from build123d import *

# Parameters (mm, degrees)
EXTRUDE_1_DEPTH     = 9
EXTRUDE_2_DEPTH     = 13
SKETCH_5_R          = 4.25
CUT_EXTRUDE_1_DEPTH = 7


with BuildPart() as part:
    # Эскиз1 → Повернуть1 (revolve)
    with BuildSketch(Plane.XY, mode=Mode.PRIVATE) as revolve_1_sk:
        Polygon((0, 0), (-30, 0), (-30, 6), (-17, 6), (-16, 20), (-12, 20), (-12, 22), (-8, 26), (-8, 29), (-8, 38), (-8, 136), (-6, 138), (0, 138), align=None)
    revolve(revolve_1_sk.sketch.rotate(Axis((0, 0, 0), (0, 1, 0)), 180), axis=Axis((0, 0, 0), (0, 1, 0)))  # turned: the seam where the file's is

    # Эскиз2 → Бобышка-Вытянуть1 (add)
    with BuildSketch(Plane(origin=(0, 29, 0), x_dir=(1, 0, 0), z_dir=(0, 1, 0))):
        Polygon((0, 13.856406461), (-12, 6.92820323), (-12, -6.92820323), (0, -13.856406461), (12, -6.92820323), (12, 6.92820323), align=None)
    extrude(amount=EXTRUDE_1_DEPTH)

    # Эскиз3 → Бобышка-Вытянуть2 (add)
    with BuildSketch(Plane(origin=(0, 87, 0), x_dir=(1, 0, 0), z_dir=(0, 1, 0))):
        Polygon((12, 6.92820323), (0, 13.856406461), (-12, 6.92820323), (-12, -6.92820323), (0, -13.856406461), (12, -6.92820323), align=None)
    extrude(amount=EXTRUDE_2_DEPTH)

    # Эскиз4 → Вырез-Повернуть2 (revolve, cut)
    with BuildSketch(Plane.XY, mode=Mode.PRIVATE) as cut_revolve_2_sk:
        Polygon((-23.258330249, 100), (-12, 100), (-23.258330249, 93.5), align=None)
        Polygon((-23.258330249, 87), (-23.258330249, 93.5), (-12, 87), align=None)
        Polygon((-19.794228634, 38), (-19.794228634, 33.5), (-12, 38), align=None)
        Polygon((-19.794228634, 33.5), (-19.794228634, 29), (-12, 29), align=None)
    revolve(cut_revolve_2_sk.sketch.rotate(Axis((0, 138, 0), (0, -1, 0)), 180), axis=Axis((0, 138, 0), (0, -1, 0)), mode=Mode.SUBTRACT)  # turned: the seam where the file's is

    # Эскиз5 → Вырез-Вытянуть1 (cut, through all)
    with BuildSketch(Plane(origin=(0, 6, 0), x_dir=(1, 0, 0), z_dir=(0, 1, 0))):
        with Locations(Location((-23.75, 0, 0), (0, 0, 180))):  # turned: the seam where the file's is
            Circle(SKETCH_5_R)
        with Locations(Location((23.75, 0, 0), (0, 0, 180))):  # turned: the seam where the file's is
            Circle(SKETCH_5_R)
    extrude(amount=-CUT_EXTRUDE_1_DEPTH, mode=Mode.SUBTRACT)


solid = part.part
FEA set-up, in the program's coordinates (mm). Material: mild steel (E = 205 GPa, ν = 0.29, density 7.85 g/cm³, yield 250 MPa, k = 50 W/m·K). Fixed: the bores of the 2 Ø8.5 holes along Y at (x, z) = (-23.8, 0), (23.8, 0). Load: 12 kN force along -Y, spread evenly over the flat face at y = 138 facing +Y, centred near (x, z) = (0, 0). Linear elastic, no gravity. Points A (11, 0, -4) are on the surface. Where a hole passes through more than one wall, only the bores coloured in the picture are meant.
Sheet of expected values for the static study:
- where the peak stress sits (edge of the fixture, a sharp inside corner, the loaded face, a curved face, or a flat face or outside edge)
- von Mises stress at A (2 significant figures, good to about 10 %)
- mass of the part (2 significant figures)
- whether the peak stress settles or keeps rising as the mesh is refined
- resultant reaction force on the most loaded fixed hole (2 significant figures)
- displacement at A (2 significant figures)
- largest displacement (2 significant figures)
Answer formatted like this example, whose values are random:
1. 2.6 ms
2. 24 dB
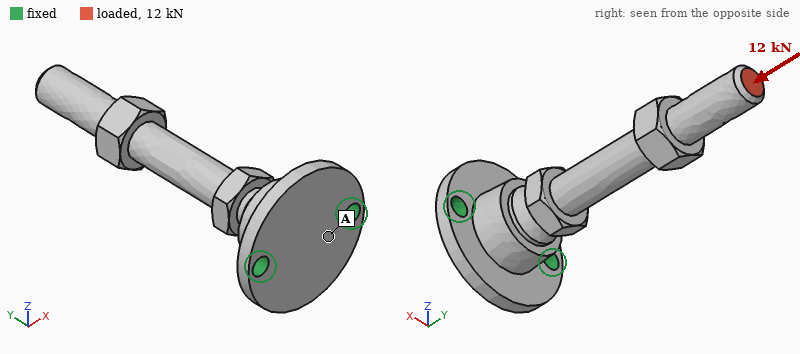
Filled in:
1. edge of the fixture
2. 35 MPa
3. 470 g
4. keeps rising
5. 6.6 kN
6. 8.7 µm
7. 44 µm
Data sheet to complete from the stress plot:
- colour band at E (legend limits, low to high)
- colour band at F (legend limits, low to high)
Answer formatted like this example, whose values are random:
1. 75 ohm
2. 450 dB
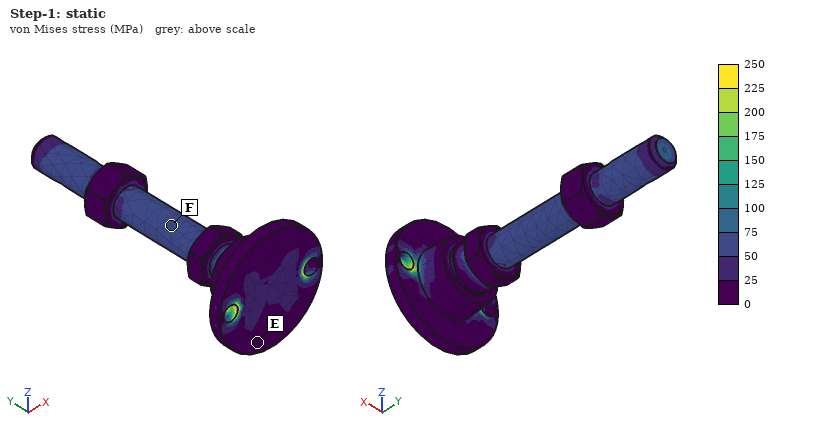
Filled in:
1. 0 to 25 MPa
2. 50 to 75 MPa
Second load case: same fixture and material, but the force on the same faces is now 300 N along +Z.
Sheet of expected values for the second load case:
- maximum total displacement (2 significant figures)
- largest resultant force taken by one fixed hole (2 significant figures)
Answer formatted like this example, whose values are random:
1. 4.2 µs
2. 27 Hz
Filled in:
1. 0.32 mm
2. 150 N
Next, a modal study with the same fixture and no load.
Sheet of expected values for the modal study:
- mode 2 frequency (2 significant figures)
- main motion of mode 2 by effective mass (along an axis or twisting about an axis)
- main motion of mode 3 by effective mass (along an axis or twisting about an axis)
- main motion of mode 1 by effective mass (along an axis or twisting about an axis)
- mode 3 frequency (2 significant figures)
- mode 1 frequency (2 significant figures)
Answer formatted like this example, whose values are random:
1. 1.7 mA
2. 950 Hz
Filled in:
1. 790 Hz
2. along X
3. along Z
4. along Z
5. 3300 Hz
6. 620 Hz
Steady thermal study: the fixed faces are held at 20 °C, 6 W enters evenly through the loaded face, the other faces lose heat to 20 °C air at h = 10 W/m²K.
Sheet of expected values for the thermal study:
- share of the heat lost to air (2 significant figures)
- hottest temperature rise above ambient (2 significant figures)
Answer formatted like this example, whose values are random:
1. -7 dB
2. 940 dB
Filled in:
1. 36 %
2. 57 K
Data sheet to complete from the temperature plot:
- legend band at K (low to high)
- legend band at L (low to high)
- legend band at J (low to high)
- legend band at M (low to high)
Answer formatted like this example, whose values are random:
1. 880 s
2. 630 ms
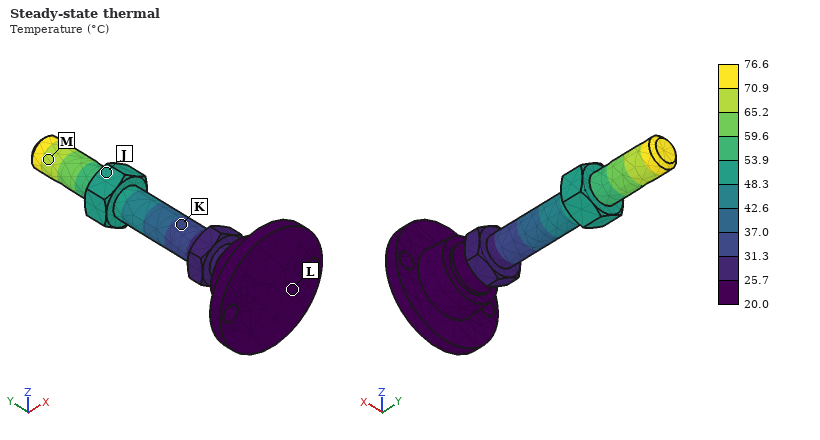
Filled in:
1. 31.3 to 37.0 °C
2. 20.0 to 25.7 °C
3. 48.3 to 53.9 °C
4. 65.2 to 70.9 °C
